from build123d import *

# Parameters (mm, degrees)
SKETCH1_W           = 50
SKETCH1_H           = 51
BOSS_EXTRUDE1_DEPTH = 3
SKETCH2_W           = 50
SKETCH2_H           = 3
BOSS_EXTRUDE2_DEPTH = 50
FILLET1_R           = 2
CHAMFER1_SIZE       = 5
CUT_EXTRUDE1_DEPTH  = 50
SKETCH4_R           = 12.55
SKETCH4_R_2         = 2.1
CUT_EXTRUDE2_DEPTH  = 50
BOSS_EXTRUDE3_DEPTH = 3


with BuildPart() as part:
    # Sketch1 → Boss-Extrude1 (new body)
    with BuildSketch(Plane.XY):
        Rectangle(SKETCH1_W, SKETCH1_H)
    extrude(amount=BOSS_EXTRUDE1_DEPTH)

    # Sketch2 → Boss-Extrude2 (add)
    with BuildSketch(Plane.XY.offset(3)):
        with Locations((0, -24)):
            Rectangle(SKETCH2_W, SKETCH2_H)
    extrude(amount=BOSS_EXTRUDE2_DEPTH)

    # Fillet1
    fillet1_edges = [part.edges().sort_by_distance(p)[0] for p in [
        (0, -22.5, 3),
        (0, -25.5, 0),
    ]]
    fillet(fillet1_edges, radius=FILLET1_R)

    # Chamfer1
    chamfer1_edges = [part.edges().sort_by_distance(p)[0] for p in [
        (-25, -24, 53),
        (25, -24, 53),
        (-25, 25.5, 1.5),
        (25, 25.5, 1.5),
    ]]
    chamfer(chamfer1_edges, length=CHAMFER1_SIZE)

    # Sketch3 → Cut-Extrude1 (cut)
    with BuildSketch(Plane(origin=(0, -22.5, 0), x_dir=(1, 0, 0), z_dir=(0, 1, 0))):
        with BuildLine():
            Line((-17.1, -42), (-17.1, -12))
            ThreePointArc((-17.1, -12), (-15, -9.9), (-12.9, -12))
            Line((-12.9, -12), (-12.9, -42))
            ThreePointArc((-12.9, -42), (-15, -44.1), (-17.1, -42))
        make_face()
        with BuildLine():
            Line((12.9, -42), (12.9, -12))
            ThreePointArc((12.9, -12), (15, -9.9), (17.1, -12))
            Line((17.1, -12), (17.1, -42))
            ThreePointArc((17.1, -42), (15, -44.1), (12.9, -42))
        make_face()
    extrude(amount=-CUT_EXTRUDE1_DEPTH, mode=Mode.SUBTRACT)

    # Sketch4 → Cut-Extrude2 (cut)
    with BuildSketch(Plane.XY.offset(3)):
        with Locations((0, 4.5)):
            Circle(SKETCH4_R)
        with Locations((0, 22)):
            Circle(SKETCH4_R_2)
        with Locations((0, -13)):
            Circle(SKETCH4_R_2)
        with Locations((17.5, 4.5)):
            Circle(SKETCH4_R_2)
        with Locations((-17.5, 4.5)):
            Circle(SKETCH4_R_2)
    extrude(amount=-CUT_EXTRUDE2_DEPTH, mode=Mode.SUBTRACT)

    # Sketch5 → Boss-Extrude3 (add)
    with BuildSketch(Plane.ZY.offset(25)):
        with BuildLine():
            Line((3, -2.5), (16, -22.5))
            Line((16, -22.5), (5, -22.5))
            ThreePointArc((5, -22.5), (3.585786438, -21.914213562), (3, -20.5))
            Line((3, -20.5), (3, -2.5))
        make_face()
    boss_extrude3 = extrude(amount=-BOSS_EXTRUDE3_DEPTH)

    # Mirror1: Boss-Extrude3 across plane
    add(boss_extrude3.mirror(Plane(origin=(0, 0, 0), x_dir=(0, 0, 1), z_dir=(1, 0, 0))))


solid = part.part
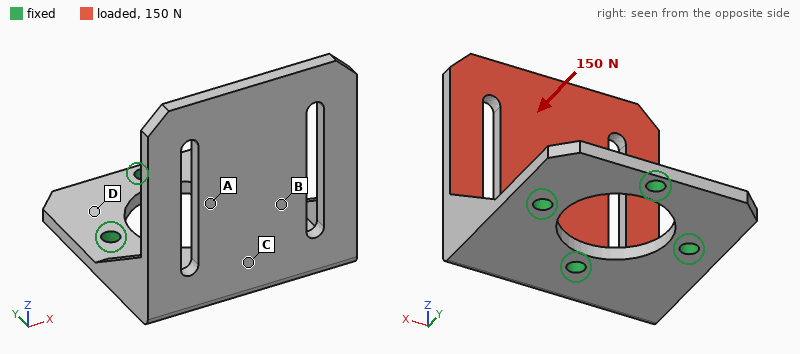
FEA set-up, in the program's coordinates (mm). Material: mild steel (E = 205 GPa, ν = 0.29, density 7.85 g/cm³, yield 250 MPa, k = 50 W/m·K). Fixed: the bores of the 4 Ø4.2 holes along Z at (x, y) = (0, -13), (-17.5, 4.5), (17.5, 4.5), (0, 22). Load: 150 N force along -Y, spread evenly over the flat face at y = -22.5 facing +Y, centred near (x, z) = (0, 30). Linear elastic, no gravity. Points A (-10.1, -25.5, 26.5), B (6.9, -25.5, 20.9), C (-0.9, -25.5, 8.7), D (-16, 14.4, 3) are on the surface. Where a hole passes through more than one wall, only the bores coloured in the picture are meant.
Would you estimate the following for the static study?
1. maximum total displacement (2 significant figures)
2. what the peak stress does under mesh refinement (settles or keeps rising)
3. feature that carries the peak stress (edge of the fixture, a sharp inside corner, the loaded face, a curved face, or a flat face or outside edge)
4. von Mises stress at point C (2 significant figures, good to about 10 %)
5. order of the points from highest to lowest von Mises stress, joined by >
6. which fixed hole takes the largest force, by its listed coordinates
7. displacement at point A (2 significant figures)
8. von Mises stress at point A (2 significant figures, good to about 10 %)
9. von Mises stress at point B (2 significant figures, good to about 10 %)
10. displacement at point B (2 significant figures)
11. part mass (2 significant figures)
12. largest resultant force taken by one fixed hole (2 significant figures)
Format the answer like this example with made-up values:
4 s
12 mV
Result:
0.13 mm
keeps rising
edge of the fixture
25 MPa
C > B > A > D
(0, -13)
0.048 mm
12 MPa
18 MPa
0.035 mm
100 g
180 N
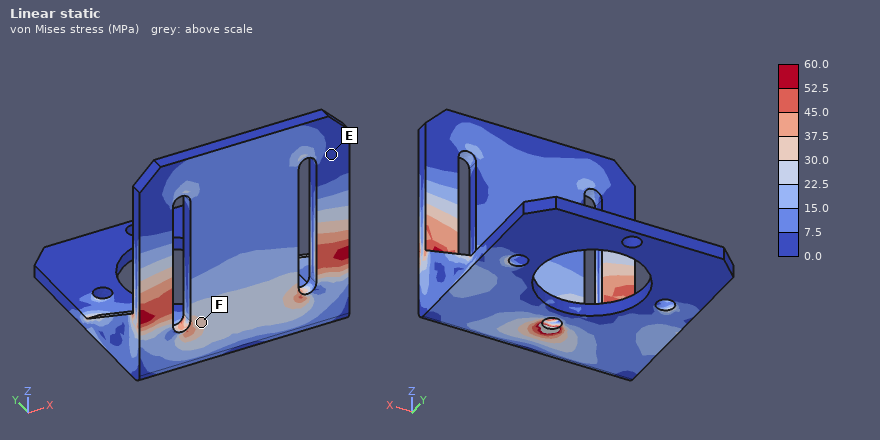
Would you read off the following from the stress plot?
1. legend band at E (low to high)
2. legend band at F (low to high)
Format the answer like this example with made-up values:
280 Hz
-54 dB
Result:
0.0 to 7.5 MPa
30.0 to 37.5 MPa
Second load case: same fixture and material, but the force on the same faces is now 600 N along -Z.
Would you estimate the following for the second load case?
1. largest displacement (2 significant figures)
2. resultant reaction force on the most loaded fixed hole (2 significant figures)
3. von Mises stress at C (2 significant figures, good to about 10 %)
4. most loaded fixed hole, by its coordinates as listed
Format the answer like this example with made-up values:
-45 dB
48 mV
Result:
28 µm
680 N
16 MPa
(0, -13)
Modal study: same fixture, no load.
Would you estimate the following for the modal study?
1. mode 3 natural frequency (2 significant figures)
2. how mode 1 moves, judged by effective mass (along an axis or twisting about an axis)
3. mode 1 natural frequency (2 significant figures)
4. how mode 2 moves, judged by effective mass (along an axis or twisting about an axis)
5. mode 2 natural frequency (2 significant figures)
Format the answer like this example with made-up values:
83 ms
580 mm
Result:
3000 Hz
along Y
980 Hz
along X
1300 Hz
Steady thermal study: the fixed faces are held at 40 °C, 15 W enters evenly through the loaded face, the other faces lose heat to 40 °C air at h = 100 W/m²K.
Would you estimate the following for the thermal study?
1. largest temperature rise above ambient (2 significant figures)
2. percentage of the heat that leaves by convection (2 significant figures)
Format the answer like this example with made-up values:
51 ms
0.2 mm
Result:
35 K
67 %
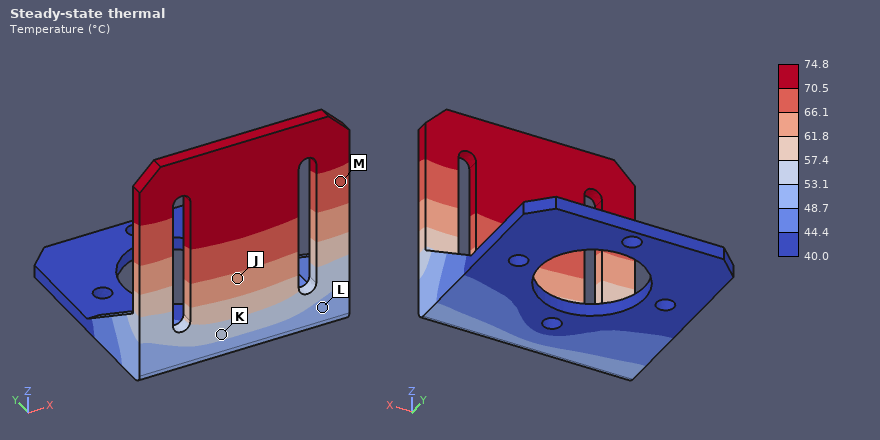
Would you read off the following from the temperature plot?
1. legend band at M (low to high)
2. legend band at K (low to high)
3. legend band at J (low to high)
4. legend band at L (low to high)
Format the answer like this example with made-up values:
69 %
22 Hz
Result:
66.1 to 70.5 °C
53.1 to 57.4 °C
61.8 to 66.1 °C
48.7 to 53.1 °C
